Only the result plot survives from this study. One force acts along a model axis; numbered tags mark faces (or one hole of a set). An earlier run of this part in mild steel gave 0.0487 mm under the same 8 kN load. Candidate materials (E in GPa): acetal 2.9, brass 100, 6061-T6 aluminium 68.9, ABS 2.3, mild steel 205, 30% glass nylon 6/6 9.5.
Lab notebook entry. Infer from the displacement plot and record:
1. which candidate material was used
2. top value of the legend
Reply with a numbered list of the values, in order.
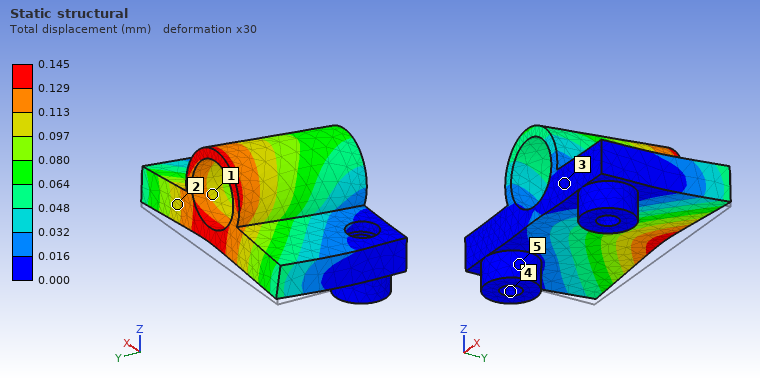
1. 6061-T6 aluminium
2. 0.145 mm
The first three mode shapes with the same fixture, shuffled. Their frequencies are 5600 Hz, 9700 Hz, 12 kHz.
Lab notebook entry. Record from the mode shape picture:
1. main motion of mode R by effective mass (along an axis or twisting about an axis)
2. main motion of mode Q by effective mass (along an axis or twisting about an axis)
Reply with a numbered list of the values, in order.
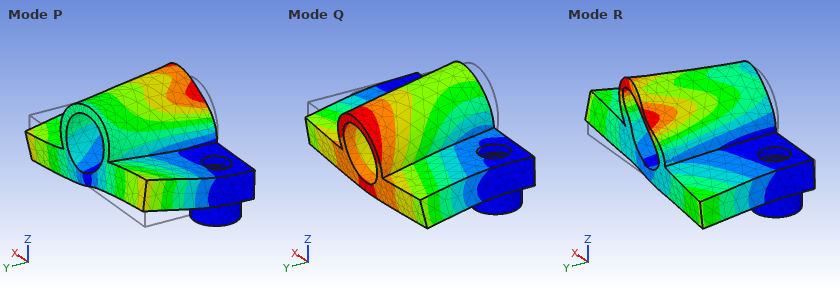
1. along X
2. along Z
